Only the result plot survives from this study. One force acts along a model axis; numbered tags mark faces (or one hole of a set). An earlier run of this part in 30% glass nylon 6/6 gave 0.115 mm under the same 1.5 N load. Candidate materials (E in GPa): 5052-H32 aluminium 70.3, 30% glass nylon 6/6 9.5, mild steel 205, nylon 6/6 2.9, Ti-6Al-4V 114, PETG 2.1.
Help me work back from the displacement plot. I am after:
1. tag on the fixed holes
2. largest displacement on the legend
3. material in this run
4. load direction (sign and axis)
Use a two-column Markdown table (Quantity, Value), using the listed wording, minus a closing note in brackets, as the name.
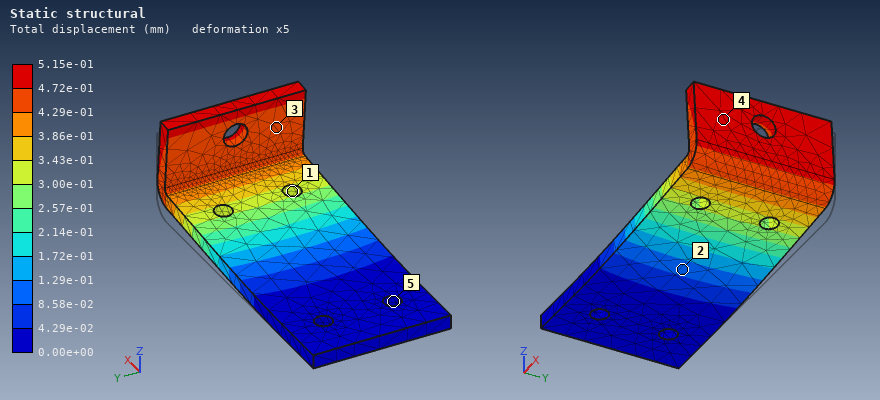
| Quantity | Value |
|---|---|
| tag on the fixed holes | 5 |
| largest displacement on the legend | 5.15e-01 mm |
| material in this run | PETG |
| load direction | +Z |
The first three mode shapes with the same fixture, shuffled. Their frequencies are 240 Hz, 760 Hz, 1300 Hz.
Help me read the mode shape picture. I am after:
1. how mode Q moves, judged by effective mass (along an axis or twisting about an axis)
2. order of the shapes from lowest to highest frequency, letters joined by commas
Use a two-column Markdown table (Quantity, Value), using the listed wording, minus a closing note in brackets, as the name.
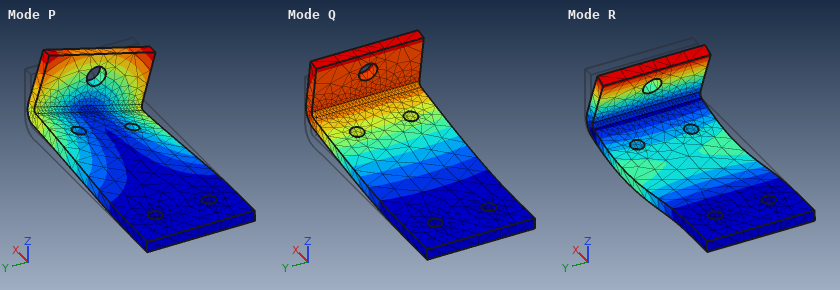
| Quantity | Value |
|---|---|
| how mode Q moves, judged by effective mass | along Z |
| order of the shapes from lowest to highest frequency, letters joined by commas | Q, P, R |
